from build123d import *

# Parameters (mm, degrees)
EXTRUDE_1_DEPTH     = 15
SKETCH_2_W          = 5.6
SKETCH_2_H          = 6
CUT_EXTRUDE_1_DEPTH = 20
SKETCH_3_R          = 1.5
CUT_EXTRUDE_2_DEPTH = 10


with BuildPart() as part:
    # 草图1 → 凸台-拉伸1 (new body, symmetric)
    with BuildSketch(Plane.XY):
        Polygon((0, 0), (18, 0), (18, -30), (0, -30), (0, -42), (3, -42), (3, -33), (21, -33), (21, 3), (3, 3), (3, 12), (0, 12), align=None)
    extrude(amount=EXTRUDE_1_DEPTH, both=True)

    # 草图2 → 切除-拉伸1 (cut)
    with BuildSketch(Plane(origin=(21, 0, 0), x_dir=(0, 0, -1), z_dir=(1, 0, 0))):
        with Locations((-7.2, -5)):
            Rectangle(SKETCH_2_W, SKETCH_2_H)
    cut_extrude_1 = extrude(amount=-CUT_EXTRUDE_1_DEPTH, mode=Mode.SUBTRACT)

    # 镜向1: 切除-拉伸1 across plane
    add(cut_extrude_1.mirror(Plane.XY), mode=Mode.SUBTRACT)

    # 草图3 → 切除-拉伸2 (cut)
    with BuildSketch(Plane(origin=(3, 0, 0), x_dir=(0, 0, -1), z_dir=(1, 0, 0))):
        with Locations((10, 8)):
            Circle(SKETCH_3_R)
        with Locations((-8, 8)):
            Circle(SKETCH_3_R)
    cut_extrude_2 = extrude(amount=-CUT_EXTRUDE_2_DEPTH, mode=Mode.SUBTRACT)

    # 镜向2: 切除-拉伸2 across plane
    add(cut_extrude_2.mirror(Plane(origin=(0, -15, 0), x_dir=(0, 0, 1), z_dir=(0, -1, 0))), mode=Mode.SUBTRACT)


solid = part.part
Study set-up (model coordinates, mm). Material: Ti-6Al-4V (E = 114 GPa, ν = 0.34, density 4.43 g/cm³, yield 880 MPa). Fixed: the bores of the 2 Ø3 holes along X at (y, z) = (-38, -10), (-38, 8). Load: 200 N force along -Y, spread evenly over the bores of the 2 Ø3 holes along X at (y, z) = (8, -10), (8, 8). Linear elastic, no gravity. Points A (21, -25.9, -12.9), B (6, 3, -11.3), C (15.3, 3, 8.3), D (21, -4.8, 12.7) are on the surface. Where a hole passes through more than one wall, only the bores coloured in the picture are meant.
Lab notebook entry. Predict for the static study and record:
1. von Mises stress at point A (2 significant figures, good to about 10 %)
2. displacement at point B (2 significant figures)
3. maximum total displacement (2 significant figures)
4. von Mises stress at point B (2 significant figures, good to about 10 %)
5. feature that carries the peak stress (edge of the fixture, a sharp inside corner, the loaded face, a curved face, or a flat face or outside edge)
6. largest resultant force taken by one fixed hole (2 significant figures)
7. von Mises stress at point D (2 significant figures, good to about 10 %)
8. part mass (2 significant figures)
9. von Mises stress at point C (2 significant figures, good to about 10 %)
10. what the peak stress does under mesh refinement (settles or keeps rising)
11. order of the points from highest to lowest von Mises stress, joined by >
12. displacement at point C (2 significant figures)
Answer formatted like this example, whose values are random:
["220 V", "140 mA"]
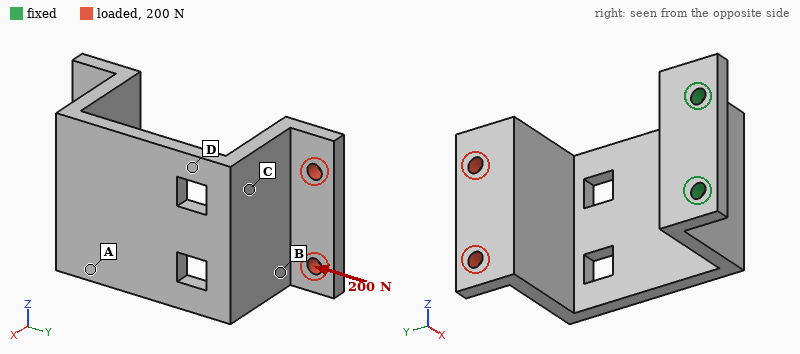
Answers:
["79 MPa", "0.50 mm", "0.76 mm", "19 MPa", "a sharp inside corner", "100 N", "120 MPa", "35 g", "50 MPa", "keeps rising", "D > A > C > B", "0.41 mm"]
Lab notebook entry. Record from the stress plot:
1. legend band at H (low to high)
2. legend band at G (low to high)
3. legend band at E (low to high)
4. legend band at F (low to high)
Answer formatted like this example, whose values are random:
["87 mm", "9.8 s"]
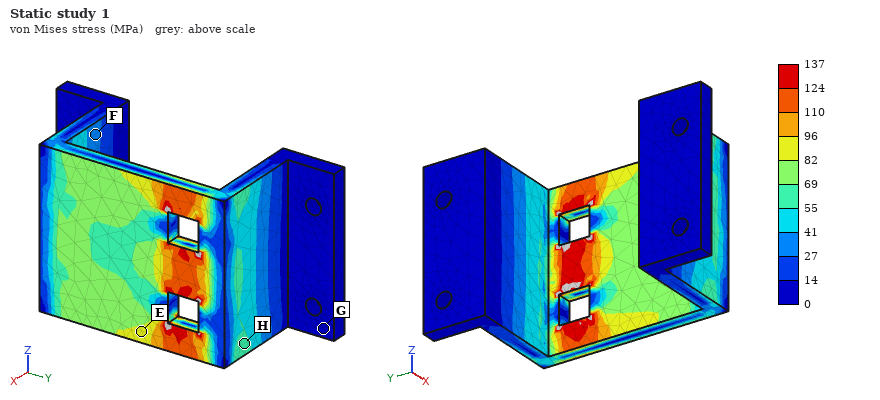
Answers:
["55 to 69 MPa", "0 to 14 MPa", "82 to 96 MPa", "27 to 41 MPa"]
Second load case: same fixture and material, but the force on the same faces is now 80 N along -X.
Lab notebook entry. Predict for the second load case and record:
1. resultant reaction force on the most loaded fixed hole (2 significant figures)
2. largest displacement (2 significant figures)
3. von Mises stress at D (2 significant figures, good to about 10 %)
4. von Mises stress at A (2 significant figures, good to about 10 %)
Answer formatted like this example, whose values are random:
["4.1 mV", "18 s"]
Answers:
["47 N", "0.70 mm", "36 MPa", "60 MPa"]
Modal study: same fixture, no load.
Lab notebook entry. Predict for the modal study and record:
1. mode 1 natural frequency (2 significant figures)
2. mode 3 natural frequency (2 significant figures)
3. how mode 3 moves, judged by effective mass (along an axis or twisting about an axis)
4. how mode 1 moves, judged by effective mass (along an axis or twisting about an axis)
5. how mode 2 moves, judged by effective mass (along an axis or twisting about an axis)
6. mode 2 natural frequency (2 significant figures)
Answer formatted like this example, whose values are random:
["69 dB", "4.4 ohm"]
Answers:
["550 Hz", "1500 Hz", "along Y", "along X", "along Z", "980 Hz"]
